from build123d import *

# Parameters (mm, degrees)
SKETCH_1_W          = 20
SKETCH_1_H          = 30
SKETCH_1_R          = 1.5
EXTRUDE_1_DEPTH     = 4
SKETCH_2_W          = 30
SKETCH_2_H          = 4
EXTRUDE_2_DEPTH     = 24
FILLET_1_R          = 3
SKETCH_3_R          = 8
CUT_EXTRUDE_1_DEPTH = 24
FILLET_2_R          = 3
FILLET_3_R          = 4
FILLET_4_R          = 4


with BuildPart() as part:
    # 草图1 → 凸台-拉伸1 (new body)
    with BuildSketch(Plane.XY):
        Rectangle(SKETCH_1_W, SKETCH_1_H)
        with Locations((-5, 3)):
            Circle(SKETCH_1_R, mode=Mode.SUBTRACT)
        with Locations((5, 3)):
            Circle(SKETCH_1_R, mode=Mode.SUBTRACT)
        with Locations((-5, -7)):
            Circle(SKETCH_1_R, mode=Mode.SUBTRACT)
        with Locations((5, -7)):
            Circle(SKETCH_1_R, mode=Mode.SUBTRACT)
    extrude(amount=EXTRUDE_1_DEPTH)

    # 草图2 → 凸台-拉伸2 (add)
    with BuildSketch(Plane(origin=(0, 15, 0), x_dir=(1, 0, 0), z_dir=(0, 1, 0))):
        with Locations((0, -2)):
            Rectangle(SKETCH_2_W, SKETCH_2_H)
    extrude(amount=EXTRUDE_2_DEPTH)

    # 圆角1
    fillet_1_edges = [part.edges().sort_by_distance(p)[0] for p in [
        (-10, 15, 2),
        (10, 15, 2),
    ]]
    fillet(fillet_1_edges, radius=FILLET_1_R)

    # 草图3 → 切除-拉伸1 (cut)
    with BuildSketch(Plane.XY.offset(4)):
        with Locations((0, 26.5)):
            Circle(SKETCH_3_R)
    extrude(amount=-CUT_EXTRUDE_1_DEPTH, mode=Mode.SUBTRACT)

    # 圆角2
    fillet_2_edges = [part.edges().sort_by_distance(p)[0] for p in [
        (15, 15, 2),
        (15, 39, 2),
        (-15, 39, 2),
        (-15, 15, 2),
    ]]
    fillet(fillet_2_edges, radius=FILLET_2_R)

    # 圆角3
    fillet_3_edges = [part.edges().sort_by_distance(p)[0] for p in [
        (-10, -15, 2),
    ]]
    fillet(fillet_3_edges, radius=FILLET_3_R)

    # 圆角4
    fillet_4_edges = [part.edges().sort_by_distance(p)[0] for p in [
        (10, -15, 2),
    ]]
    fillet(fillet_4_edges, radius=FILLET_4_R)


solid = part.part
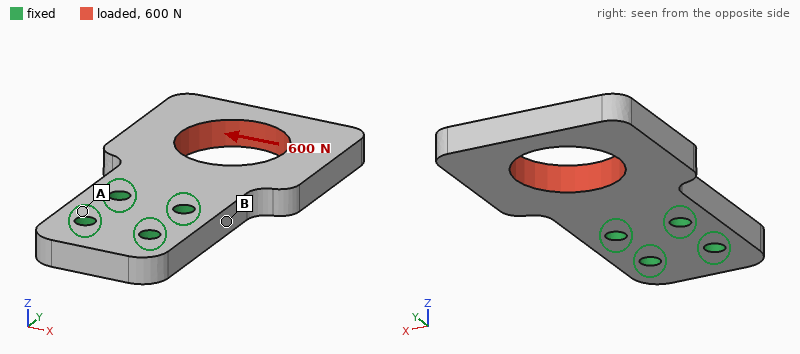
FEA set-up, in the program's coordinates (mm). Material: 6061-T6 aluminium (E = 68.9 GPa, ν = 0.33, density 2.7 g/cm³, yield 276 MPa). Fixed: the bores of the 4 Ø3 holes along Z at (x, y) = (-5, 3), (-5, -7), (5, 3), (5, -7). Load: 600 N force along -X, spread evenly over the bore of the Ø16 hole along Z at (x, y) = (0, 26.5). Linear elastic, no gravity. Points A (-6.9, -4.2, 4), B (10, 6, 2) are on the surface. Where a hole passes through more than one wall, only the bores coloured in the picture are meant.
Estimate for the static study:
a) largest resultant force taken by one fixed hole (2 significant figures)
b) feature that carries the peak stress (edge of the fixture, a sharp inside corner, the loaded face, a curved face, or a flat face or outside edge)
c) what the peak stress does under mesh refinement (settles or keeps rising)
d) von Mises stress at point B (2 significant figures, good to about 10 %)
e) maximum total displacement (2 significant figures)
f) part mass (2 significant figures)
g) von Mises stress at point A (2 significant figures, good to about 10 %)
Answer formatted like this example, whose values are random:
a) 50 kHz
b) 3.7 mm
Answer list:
a) 990 N
b) edge of the fixture
c) keeps rising
d) 37 MPa
e) 58 µm
f) 12 g
g) 9.2 MPa
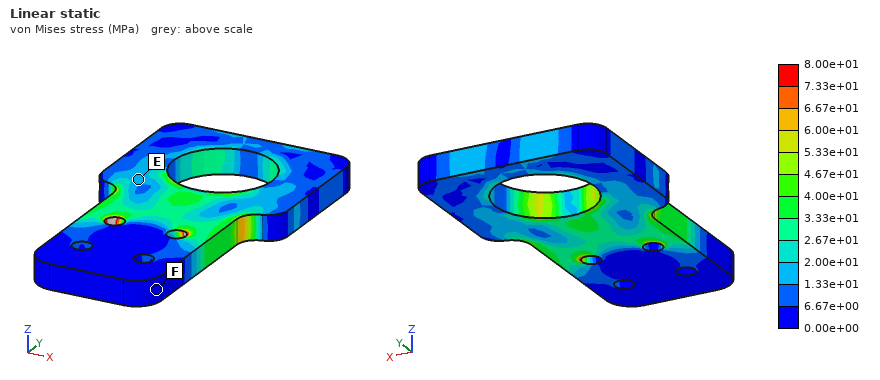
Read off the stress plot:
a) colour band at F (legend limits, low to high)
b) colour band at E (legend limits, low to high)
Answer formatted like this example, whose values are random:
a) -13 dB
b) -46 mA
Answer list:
a) 0.00e+00 to 6.67e+00 MPa
b) 1.33e+01 to 2.00e+01 MPa
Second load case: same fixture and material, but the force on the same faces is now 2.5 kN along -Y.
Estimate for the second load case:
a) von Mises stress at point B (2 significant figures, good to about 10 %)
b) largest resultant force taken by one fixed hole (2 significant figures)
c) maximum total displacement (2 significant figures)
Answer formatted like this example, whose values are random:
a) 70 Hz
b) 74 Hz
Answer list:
a) 25 MPa
b) 1.1 kN
c) 33 µm
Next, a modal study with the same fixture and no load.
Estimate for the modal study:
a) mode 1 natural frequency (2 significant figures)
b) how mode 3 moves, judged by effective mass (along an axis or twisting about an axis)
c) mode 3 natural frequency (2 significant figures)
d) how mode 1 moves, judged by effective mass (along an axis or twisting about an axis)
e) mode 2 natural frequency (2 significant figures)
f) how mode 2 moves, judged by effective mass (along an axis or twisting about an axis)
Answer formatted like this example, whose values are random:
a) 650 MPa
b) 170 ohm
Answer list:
a) 2300 Hz
b) along X
c) 7600 Hz
d) along Z
e) 5000 Hz
f) twisting about Y
